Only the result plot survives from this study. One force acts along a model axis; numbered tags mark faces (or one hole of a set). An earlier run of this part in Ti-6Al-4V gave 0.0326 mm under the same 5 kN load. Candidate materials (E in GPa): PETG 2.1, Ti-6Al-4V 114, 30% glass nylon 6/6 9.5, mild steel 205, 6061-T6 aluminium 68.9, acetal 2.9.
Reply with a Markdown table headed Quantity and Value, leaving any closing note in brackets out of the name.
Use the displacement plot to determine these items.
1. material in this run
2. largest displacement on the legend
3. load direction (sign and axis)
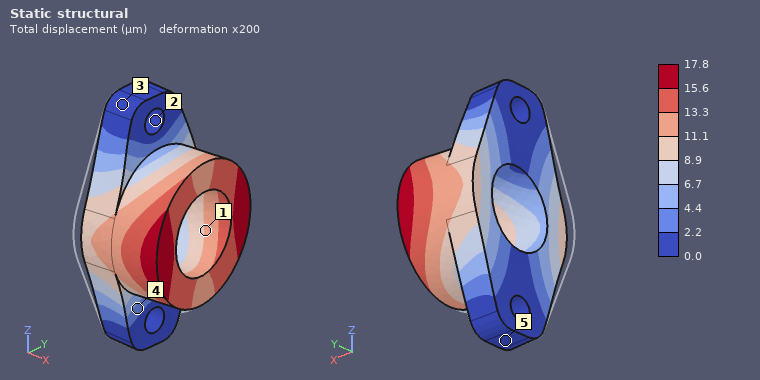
| Quantity | Value |
|---|---|
| material in this run | mild steel |
| largest displacement on the legend | 17.8 µm |
| load direction | +Y |
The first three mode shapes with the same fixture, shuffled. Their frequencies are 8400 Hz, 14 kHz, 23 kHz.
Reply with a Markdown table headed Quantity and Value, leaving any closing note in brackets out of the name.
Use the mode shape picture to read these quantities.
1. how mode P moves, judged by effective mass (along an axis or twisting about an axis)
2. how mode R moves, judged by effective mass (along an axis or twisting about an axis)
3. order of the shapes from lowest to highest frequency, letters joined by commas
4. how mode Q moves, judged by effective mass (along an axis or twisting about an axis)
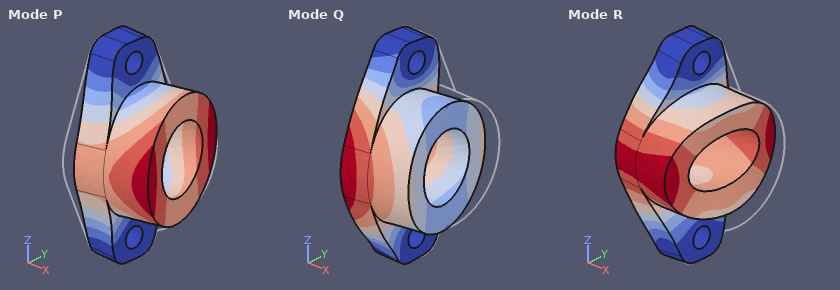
| Quantity | Value |
|---|---|
| how mode P moves, judged by effective mass | along Y |
| how mode R moves, judged by effective mass | along X |
| order of the shapes from lowest to highest frequency, letters joined by commas | P, R, Q |
| how mode Q moves, judged by effective mass | along Y |
